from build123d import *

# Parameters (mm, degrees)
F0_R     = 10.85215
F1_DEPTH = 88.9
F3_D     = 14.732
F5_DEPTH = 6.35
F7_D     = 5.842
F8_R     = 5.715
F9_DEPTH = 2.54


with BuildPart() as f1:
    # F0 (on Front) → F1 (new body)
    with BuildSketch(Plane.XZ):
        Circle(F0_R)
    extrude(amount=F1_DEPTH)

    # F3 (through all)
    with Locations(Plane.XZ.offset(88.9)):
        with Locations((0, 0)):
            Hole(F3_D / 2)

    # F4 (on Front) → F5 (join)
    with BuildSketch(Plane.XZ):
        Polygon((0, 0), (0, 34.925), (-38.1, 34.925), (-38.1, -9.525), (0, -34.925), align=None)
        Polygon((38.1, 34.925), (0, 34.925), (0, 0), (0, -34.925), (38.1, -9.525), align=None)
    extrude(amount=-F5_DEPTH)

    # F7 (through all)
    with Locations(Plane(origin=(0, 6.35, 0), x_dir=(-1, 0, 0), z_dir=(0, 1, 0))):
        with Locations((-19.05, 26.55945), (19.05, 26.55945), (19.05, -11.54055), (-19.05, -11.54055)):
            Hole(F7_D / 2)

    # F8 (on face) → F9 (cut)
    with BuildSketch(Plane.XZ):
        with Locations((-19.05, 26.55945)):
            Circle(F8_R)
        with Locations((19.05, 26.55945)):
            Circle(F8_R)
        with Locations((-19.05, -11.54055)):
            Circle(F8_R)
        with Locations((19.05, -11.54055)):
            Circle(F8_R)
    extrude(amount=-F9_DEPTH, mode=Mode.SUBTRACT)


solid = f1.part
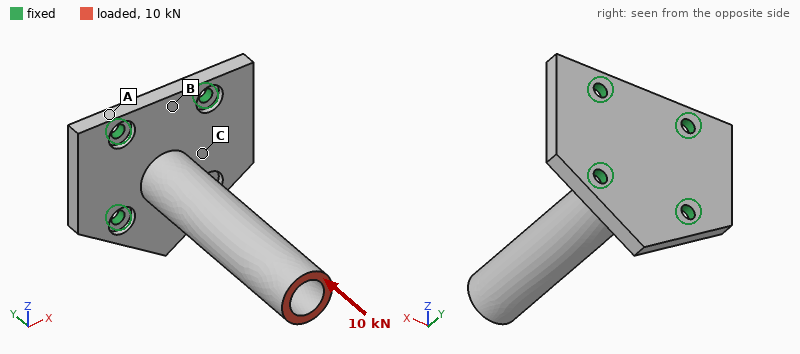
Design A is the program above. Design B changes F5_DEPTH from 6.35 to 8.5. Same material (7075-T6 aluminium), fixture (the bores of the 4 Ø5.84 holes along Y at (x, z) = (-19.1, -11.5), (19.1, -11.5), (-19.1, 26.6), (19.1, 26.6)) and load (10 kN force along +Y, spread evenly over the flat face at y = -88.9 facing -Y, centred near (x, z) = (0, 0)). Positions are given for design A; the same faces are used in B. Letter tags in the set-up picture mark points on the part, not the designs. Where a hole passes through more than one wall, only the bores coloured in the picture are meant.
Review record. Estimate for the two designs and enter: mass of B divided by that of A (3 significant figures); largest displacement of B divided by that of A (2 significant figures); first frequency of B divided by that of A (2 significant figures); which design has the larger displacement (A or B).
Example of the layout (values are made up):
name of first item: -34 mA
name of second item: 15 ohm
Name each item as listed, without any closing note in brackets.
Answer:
mass of B divided by that of A: 1.21
largest displacement of B divided by that of A: 0.64
first frequency of B divided by that of A: 1.1
which design has the larger displacement: A
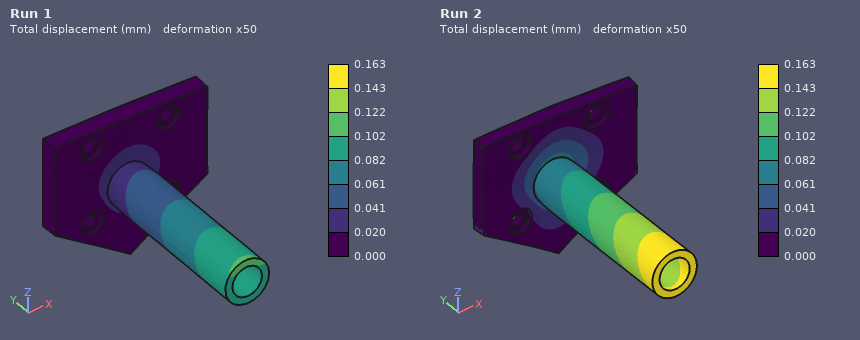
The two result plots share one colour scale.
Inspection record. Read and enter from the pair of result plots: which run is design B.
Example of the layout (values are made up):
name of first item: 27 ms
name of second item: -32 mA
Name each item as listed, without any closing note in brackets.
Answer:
which run is design B: Run 1
